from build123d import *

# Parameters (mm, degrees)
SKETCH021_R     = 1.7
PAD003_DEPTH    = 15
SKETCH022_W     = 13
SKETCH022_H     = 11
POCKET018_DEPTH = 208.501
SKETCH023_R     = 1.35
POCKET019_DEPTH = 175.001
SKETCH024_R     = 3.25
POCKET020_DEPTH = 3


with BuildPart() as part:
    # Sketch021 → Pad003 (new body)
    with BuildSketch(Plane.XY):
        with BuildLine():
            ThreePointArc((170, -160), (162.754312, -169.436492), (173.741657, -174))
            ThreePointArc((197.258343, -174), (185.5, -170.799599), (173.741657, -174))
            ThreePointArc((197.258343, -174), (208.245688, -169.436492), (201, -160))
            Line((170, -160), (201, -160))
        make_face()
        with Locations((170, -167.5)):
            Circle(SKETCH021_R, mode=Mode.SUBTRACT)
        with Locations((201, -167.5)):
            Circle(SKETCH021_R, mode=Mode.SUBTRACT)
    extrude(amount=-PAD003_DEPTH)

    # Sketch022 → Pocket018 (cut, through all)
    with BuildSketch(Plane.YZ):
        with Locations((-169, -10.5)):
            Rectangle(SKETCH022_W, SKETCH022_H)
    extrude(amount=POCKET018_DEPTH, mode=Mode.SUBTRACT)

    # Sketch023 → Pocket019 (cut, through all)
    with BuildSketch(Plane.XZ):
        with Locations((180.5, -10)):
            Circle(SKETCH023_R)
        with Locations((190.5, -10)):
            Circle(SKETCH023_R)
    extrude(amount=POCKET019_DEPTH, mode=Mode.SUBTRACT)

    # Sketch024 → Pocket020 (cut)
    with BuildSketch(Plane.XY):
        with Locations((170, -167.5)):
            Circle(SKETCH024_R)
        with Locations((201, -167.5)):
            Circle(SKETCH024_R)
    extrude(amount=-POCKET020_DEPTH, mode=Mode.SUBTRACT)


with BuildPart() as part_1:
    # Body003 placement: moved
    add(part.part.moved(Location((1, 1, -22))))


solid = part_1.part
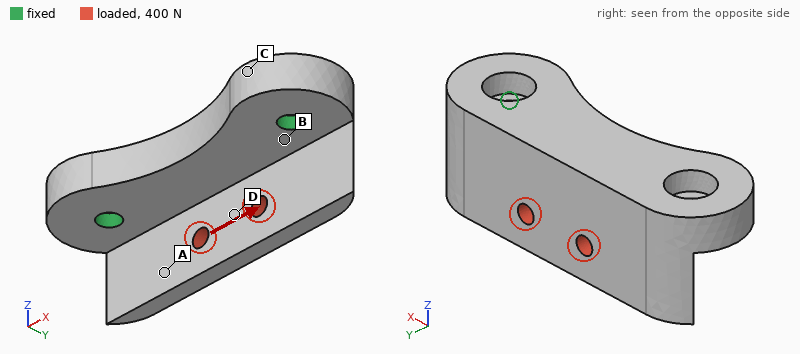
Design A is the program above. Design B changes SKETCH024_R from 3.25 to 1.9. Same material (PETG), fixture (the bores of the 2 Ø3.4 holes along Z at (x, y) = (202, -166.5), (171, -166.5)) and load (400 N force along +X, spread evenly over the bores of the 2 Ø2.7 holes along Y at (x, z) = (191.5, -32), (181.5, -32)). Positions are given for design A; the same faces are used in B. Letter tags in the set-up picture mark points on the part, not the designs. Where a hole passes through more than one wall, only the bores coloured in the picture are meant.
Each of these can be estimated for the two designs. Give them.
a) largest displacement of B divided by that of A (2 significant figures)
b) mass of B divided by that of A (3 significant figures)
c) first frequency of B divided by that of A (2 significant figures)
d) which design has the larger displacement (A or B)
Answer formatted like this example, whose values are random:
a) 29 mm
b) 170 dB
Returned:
a) 0.86
b) 1.04
c) 1.1
d) A
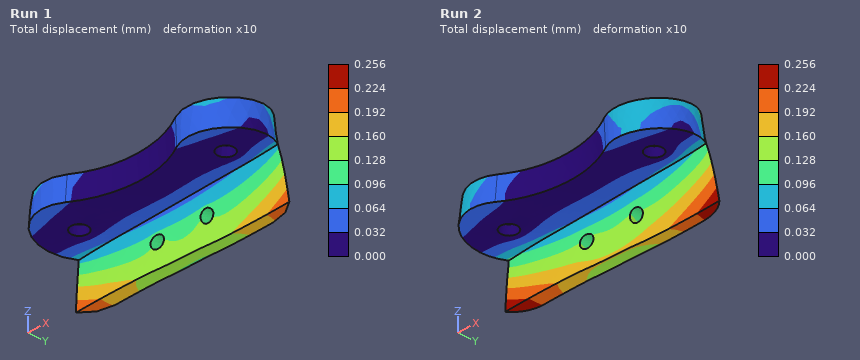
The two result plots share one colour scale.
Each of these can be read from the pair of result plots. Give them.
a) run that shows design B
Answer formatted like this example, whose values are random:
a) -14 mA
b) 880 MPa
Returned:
a) Run 1
